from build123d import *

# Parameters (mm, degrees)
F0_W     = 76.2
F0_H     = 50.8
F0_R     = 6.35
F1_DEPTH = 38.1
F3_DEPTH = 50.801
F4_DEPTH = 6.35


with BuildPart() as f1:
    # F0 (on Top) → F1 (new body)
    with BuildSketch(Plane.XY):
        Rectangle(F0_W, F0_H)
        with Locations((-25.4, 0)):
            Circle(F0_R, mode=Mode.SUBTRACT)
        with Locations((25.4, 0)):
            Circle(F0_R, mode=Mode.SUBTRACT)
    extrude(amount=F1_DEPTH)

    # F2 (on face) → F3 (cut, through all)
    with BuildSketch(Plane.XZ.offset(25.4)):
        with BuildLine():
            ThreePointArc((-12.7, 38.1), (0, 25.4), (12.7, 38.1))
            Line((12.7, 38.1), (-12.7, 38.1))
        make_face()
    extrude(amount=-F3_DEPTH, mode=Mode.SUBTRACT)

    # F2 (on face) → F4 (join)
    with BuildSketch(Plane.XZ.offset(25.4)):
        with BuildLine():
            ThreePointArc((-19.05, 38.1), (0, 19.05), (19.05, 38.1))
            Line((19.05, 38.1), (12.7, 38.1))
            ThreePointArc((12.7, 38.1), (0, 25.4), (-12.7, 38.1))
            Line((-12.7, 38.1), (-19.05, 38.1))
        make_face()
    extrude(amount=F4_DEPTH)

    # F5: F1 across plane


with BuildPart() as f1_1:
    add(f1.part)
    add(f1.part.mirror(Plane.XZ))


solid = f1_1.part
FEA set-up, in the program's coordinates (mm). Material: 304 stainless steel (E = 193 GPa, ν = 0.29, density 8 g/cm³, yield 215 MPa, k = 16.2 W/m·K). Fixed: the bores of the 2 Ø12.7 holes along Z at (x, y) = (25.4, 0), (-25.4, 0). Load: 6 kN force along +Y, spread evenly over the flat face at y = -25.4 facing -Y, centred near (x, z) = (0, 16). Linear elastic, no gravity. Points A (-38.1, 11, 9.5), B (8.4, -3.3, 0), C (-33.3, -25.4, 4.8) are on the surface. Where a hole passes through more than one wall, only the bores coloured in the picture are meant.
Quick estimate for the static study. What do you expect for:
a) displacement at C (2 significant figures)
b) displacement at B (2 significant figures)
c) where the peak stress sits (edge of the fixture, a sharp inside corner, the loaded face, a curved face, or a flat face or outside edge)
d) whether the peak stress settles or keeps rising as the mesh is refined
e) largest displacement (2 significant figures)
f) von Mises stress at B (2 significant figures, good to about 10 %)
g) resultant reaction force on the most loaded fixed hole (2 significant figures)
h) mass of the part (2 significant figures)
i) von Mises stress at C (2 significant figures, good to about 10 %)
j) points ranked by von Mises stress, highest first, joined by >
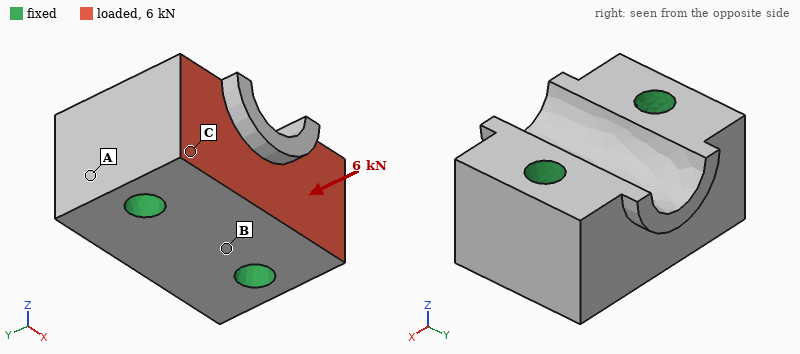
0.35 µm
0.23 µm
edge of the fixture
keeps rising
0.52 µm
1.5 MPa
3.0 kN
1.0 kg
2.7 MPa
C > B > A
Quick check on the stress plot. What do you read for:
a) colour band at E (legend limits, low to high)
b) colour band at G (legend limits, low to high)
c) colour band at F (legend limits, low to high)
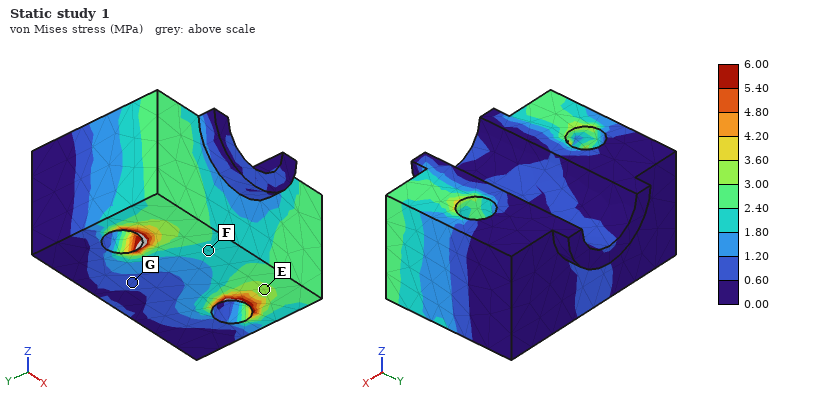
3.00 to 3.60 MPa
0.60 to 1.20 MPa
1.80 to 2.40 MPa
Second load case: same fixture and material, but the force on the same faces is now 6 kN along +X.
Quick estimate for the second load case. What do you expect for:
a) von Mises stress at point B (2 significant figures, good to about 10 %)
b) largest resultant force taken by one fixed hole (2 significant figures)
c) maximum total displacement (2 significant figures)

3.2 MPa
3.6 kN
1.6 µm
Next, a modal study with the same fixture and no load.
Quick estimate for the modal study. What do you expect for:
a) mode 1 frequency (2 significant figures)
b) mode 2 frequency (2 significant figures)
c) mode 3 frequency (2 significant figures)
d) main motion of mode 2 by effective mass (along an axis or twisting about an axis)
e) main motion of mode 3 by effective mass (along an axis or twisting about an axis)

22 kHz
23 kHz
25 kHz
along Z
twisting about Z
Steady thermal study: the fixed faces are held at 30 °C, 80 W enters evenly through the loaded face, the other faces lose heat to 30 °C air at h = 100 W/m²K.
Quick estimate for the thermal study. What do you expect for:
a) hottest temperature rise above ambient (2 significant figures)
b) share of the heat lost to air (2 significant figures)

44 K
18 %
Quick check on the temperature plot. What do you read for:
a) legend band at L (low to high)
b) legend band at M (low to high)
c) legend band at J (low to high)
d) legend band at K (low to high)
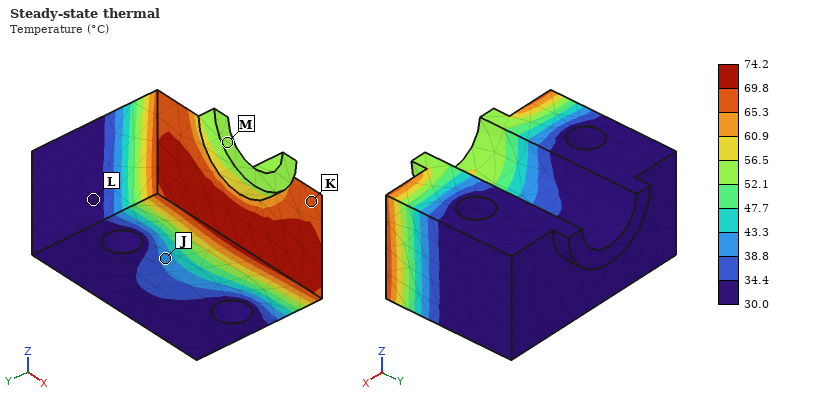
30.0 to 34.4 °C
52.1 to 56.5 °C
38.8 to 43.3 °C
65.3 to 69.8 °C
